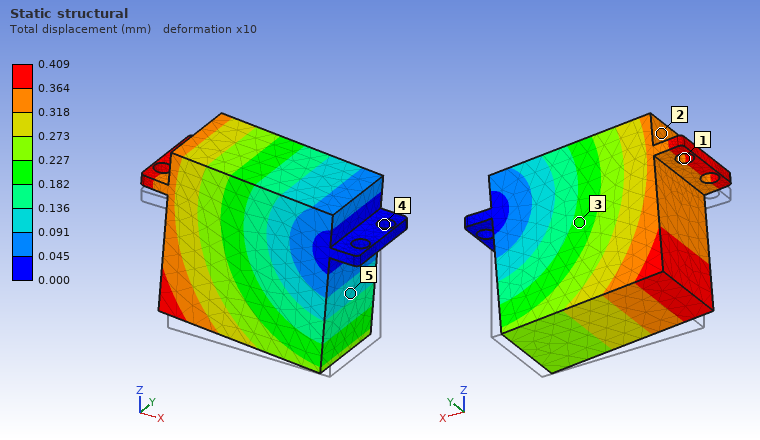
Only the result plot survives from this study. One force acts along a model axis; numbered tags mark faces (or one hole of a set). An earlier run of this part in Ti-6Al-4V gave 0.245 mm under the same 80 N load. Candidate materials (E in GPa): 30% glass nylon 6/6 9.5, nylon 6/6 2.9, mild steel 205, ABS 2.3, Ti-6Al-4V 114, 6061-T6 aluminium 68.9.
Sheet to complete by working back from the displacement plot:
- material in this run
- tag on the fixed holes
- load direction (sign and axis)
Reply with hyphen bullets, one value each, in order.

- 6061-T6 aluminium
- 4
- +Z
